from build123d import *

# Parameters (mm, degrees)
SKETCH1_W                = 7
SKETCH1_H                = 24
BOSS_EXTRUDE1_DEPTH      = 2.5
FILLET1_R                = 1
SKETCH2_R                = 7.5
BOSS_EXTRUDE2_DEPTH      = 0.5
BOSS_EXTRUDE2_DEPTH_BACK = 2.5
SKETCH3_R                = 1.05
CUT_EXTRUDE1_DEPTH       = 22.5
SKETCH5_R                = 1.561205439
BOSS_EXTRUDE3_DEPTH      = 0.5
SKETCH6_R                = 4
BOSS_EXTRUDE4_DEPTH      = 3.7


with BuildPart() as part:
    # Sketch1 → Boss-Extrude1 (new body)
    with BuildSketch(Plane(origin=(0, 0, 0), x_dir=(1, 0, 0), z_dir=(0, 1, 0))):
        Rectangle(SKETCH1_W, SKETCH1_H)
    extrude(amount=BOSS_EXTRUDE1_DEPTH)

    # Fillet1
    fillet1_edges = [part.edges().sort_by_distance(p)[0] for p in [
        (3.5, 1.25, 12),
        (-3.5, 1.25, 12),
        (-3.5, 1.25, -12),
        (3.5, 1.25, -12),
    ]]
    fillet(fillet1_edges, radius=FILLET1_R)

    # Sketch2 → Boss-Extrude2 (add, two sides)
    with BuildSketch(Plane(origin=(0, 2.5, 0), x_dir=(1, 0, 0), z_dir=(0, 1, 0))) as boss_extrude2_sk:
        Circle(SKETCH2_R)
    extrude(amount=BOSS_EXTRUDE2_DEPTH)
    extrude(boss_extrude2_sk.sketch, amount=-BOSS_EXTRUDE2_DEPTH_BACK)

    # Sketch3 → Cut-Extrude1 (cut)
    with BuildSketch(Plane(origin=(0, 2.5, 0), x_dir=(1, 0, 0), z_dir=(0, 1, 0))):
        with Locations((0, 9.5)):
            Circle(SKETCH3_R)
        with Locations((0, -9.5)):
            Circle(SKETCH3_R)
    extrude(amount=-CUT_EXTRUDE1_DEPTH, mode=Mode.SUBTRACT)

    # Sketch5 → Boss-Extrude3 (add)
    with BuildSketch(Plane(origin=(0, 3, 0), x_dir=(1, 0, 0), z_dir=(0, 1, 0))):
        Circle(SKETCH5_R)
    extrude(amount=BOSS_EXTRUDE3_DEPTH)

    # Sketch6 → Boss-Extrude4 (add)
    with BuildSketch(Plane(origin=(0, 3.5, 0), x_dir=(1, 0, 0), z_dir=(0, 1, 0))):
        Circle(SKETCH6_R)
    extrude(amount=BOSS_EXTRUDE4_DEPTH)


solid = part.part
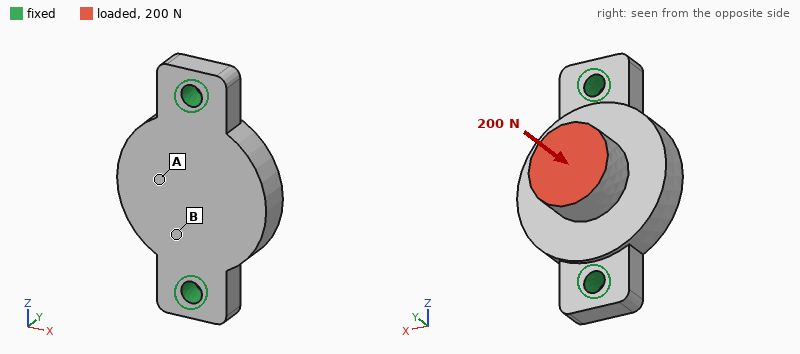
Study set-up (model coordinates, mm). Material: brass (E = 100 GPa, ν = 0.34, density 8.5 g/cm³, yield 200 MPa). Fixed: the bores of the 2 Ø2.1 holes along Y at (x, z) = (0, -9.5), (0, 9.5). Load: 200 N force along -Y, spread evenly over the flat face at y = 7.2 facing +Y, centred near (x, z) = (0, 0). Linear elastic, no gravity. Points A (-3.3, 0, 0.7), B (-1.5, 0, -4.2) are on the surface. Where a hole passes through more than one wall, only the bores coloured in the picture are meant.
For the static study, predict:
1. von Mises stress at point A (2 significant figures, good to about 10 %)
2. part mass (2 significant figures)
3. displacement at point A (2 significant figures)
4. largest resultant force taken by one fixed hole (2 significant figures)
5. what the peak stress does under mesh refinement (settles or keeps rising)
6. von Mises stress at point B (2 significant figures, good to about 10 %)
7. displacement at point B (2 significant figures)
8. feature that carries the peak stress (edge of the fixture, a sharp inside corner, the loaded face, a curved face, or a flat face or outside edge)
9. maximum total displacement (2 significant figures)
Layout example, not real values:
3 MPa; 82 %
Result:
19 MPa; 7.4 g; 4.2 µm; 110 N; keeps rising; 8.3 MPa; 3.0 µm; edge of the fixture; 5.2 µm
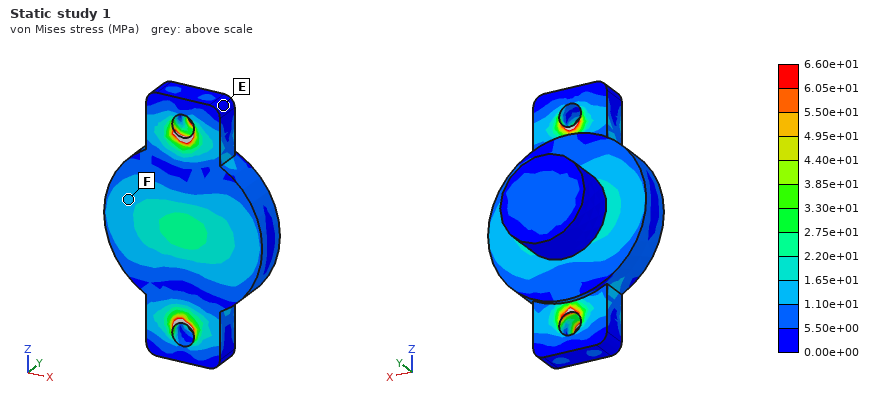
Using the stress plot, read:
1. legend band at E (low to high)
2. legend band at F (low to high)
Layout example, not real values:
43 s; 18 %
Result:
0.00e+00 to 5.50e+00 MPa; 1.10e+01 to 1.65e+01 MPa
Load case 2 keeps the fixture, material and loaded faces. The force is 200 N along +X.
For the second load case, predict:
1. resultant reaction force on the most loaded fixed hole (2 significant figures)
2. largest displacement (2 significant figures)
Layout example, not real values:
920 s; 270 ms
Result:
100 N; 35 µm
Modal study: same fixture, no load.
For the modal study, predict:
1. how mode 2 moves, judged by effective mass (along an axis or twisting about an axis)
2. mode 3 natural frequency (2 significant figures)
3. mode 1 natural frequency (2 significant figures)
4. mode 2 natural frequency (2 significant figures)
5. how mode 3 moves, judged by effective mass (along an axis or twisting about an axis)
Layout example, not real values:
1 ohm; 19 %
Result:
along Y; 18 kHz; 11 kHz; 15 kHz; along Z
